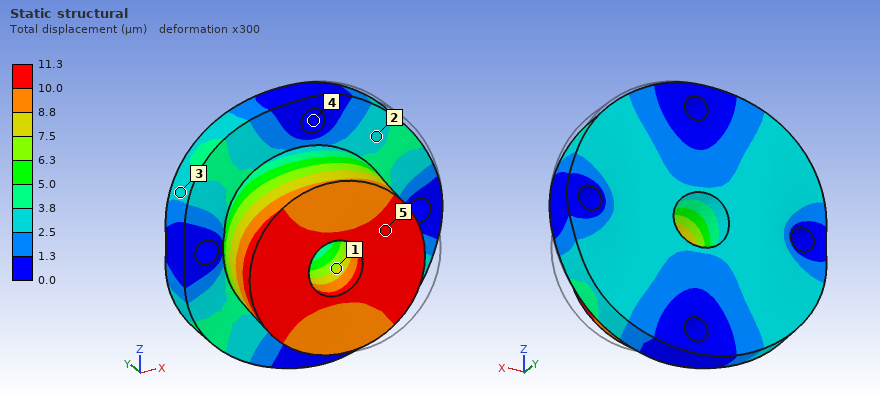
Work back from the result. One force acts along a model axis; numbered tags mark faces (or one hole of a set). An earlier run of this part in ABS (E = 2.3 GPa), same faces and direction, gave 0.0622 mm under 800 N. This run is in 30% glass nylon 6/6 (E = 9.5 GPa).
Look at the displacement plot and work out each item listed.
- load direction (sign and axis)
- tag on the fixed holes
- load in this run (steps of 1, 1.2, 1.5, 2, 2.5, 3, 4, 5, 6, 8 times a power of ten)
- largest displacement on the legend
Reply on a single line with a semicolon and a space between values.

-X; 4; 600 N; 11.3 µm
